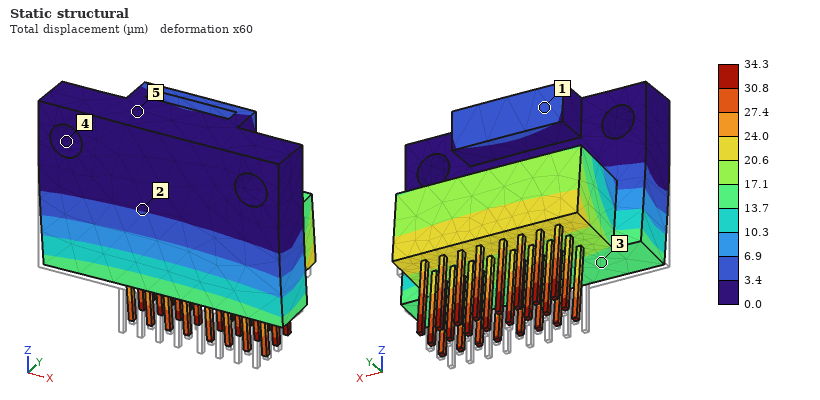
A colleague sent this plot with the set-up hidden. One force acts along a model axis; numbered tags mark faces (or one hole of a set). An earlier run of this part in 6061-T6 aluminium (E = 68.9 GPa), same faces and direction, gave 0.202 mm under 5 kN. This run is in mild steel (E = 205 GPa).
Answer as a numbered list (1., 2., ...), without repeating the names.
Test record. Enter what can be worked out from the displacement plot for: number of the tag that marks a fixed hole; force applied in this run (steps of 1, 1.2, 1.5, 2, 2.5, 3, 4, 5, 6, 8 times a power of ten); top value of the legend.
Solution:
1. 4
2. 2.5 kN
3. 34.3 µm
